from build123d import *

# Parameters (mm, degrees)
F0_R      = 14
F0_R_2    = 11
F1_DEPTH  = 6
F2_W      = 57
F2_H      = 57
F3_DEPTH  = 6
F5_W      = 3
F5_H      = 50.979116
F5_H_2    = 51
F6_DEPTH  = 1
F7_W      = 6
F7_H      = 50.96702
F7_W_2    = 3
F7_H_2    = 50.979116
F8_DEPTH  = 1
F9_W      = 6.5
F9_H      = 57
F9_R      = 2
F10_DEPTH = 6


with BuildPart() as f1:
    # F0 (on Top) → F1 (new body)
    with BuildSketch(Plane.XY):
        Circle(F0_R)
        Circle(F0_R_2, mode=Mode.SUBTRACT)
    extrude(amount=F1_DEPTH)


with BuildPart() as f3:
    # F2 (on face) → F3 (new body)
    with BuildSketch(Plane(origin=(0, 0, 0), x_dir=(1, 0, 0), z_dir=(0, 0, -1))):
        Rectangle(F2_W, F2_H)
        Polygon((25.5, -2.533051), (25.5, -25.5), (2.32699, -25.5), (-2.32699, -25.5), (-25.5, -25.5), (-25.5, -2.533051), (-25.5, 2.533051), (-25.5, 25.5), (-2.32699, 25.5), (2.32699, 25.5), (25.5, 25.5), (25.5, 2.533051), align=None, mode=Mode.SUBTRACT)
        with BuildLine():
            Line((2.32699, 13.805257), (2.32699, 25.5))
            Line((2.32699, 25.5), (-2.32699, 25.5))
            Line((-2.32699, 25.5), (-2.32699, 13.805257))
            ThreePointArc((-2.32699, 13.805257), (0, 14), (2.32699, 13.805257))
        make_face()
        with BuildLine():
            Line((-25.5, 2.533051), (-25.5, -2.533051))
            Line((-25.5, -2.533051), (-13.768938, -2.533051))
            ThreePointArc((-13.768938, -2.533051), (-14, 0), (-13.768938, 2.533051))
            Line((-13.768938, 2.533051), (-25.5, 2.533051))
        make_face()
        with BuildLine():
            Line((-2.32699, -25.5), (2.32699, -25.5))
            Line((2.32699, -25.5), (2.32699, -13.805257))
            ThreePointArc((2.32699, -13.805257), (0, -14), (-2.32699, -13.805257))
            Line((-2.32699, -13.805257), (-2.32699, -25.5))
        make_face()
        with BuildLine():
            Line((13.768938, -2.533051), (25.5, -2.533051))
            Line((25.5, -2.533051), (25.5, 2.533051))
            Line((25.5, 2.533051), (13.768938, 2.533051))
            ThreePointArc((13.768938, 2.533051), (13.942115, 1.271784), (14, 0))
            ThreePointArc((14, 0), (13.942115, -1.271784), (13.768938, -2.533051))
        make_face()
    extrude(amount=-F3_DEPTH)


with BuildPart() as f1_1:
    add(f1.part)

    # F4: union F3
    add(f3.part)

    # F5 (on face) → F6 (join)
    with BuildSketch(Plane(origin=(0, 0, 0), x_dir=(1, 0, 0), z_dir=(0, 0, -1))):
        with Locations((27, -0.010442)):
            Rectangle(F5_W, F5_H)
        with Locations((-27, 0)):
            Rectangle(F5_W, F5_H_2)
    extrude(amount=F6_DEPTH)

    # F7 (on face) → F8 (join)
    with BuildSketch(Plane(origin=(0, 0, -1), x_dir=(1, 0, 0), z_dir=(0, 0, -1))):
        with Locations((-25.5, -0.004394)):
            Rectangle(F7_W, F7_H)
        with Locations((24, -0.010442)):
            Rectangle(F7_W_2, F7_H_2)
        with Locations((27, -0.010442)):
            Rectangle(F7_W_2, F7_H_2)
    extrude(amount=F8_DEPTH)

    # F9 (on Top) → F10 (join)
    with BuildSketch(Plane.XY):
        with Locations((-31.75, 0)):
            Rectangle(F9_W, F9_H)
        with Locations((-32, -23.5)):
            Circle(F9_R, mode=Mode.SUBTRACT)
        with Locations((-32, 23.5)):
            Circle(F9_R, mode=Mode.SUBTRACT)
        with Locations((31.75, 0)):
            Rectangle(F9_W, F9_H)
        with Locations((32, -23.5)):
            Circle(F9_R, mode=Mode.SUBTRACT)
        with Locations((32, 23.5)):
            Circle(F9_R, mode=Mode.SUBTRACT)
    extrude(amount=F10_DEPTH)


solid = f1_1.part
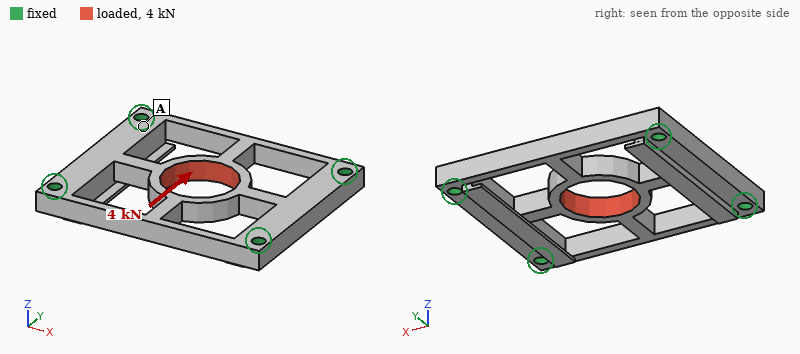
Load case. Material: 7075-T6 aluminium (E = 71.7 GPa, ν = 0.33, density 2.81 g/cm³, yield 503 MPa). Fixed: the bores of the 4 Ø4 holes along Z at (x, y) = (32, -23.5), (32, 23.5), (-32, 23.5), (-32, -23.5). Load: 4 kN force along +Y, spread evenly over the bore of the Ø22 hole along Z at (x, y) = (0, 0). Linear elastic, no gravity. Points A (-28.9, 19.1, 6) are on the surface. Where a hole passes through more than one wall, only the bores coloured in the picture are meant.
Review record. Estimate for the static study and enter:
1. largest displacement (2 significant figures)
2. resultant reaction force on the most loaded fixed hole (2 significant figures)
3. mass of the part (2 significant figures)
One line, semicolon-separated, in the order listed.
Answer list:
0.21 mm; 1.2 kN; 33 g
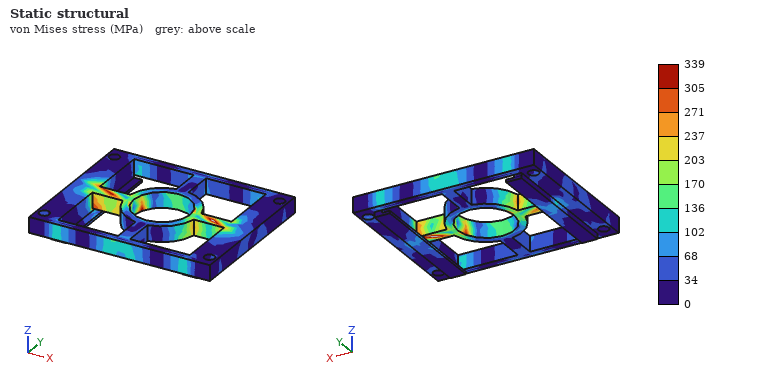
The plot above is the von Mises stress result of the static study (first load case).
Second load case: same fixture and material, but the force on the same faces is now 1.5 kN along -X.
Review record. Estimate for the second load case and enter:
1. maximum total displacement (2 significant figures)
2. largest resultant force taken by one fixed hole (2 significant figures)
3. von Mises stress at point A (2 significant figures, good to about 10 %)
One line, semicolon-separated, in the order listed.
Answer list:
40 µm; 440 N; 13 MPa
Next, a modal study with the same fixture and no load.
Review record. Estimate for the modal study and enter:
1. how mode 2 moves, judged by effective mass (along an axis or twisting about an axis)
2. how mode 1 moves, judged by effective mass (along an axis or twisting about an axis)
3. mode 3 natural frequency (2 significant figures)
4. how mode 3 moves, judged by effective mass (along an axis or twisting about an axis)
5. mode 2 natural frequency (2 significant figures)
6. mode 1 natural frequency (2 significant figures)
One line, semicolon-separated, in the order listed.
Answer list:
twisting about X; along Z; 8000 Hz; along Y; 7100 Hz; 5500 Hz
